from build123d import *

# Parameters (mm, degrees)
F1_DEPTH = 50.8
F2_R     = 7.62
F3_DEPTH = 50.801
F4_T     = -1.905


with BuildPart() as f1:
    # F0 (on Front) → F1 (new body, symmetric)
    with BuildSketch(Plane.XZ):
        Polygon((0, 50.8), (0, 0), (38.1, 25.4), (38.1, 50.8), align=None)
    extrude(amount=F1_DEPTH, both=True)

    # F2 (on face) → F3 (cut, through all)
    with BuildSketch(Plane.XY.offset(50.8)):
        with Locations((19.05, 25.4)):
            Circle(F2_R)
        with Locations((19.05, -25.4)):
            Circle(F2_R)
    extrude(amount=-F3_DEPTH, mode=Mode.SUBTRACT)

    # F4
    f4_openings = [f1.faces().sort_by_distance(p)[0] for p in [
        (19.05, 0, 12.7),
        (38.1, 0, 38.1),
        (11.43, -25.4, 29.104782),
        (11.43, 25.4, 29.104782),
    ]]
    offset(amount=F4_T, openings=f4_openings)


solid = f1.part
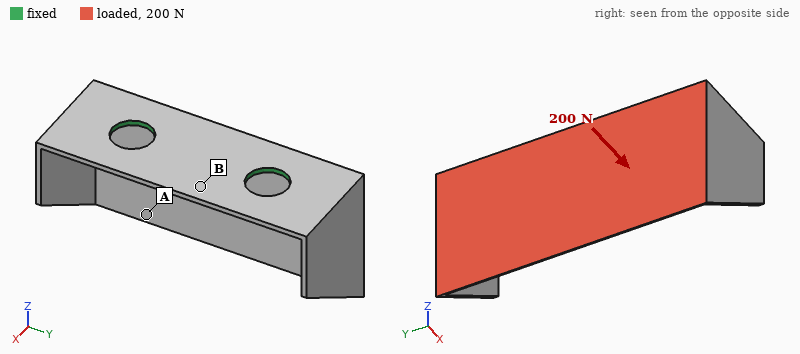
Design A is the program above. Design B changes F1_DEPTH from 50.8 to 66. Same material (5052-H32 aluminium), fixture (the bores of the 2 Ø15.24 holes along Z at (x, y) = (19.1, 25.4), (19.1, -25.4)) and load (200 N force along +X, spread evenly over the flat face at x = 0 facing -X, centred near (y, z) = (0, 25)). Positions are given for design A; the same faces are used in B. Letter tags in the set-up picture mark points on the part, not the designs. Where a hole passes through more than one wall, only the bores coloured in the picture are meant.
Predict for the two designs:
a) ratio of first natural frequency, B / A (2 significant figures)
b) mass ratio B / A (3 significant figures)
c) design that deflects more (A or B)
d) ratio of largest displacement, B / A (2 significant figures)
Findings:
0.74
1.24
B
1.3
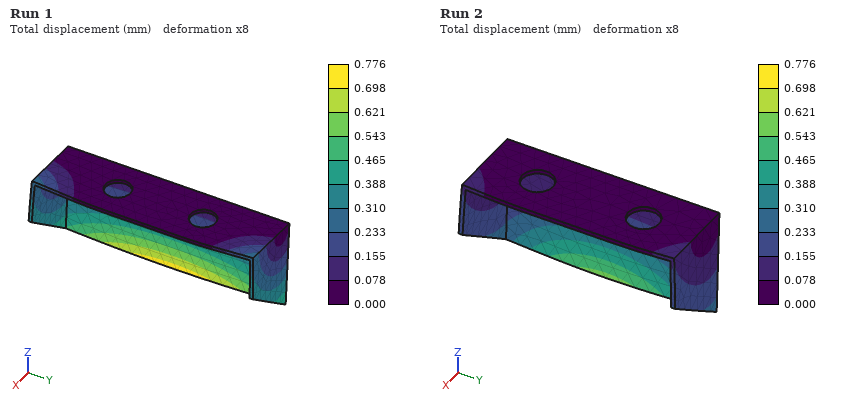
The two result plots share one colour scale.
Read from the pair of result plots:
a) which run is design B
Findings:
Run 1
